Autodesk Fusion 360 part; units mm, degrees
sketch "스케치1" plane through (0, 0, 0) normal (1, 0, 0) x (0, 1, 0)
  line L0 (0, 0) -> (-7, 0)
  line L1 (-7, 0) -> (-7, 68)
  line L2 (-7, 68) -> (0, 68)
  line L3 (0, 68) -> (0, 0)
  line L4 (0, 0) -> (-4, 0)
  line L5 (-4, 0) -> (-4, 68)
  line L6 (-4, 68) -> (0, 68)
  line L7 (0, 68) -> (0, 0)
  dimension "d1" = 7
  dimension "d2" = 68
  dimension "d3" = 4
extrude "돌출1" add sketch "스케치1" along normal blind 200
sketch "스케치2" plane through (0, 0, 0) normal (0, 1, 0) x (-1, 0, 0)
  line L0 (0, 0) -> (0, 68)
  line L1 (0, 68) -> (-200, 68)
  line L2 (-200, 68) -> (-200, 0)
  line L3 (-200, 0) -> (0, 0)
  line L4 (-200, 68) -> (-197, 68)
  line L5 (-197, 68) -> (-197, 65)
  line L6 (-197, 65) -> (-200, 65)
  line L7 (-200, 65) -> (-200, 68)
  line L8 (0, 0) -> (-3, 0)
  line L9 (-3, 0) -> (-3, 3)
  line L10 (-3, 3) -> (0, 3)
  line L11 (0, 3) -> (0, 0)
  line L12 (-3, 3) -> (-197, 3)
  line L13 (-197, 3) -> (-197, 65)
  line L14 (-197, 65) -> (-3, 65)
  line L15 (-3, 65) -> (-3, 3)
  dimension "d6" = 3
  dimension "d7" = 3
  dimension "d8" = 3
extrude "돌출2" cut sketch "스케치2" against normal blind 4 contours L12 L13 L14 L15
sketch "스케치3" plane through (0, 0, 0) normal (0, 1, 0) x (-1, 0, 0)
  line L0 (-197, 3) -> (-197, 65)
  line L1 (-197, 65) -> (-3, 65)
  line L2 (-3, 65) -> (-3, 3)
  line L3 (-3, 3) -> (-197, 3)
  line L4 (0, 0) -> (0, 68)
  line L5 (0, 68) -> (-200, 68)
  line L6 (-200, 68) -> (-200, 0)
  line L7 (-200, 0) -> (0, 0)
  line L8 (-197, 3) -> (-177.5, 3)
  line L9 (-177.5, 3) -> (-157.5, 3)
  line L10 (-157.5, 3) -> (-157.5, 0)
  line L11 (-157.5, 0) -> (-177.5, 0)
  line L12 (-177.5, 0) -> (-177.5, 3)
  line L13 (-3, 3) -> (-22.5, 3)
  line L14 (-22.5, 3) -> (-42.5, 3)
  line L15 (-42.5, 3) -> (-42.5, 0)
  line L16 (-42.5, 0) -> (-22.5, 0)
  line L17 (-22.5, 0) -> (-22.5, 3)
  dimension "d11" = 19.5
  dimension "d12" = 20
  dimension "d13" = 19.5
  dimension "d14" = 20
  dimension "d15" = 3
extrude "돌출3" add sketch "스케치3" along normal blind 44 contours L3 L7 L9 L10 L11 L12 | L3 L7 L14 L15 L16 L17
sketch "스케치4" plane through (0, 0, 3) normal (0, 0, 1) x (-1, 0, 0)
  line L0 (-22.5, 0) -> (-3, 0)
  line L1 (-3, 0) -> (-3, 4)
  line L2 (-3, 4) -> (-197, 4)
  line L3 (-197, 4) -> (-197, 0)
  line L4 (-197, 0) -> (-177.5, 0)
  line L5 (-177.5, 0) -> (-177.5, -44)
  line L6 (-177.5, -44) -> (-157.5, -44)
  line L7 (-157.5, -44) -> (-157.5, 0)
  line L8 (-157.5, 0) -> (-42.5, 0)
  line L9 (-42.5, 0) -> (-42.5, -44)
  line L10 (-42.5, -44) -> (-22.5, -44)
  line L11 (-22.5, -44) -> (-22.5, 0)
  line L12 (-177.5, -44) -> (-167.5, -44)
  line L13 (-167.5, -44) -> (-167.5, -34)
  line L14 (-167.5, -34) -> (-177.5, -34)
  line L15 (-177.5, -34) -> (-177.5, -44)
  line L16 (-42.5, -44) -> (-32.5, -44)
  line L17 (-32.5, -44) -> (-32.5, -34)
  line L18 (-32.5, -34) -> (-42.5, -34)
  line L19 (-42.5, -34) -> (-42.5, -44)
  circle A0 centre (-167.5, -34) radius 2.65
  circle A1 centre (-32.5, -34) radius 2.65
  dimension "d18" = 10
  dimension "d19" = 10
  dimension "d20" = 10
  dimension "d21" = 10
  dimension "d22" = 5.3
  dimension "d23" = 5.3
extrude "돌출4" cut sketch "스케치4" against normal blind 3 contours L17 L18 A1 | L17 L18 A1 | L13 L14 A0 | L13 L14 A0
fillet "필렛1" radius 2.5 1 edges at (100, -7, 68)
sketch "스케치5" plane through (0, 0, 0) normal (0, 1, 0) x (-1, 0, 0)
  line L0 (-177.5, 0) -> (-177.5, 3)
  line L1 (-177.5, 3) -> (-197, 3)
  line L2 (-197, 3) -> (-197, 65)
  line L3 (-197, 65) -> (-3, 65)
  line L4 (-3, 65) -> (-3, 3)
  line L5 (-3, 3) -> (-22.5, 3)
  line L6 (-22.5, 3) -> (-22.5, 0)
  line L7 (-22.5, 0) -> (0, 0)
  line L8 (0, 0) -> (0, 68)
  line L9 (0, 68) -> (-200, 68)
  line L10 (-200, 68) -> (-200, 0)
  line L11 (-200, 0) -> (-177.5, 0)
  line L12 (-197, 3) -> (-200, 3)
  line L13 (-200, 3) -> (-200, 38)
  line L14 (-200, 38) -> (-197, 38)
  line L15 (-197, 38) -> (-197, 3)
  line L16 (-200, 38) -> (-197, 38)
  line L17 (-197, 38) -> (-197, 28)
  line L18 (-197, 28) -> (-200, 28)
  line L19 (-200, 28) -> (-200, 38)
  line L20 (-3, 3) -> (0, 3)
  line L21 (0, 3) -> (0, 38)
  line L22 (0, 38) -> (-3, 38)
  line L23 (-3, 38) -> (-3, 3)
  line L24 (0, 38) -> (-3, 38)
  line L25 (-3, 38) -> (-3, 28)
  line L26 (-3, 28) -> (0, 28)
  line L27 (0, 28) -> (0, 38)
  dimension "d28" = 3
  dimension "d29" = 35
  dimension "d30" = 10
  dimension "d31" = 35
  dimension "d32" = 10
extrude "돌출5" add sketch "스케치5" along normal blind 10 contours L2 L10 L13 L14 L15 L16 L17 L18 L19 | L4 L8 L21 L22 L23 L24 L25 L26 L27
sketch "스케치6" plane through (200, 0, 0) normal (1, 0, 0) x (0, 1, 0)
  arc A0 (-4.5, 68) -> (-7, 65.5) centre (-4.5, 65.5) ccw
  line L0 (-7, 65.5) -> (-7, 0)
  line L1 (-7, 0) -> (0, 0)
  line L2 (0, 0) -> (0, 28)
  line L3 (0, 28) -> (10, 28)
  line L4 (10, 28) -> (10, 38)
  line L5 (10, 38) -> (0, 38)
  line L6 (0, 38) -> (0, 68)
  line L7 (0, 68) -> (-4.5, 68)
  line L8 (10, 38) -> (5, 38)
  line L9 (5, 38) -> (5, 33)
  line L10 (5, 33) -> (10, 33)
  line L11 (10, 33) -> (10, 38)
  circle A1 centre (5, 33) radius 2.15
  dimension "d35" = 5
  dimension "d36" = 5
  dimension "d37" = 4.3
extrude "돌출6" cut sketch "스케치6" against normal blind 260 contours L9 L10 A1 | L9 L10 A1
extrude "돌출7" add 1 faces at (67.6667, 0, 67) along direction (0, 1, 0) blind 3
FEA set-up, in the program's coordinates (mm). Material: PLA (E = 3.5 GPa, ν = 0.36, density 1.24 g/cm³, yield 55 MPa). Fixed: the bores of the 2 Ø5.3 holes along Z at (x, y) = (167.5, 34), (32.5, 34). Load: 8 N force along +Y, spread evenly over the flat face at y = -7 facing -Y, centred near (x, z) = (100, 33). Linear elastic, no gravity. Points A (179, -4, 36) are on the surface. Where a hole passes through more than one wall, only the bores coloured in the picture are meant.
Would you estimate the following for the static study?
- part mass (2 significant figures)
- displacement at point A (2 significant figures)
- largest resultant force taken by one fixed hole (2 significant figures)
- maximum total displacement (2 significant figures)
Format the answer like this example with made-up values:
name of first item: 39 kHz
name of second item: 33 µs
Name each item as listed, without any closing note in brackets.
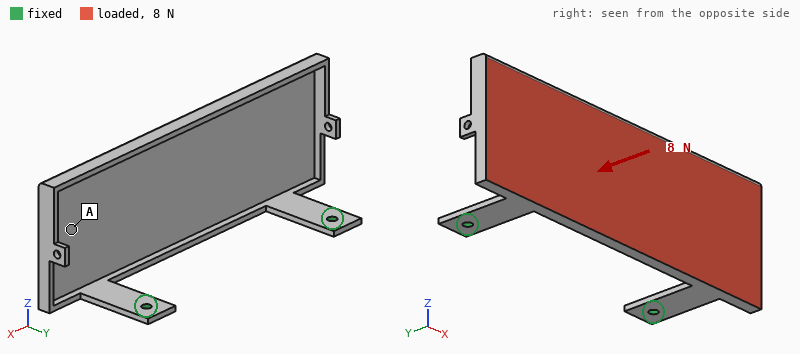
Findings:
part mass: 68 g
displacement at point A: 1.2 mm
largest resultant force taken by one fixed hole: 4.1 N
maximum total displacement: 2.2 mm
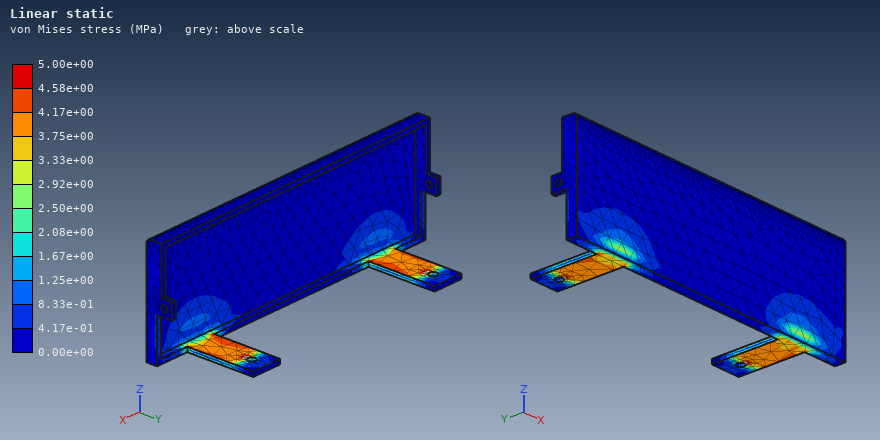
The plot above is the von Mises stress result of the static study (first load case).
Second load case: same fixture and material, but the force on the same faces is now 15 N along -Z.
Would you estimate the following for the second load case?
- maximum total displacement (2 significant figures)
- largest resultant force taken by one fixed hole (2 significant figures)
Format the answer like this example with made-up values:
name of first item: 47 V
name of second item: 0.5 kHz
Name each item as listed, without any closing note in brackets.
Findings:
maximum total displacement: 2.6 mm
largest resultant force taken by one fixed hole: 7.5 N
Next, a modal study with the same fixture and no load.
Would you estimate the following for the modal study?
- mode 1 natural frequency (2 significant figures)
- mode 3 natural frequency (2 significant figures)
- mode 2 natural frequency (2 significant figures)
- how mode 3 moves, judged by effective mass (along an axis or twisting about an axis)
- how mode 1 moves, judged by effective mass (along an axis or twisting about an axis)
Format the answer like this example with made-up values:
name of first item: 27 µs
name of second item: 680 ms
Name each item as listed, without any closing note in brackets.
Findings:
mode 1 natural frequency: 41 Hz
mode 3 natural frequency: 160 Hz
mode 2 natural frequency: 100 Hz
how mode 3 moves, judged by effective mass: along Z
how mode 1 moves, judged by effective mass: along Y
